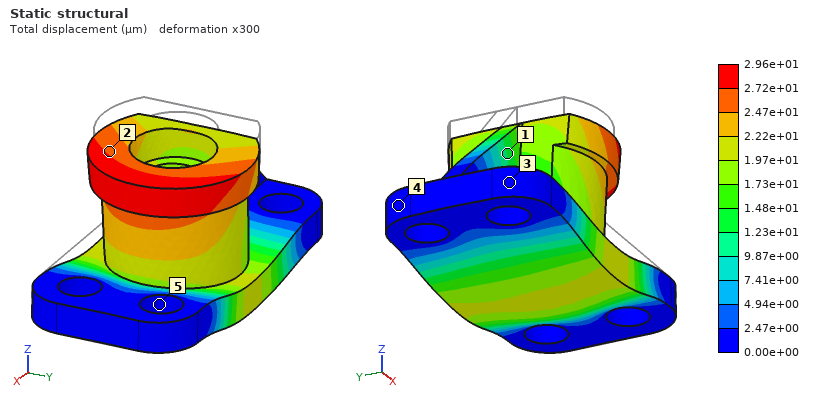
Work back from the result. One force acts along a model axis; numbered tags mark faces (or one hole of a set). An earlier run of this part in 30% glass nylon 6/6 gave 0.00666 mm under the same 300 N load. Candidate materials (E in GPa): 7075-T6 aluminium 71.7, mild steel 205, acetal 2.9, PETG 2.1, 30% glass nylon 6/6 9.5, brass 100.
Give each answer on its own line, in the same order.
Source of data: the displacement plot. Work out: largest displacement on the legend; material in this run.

2.96e+01 µm
PETG
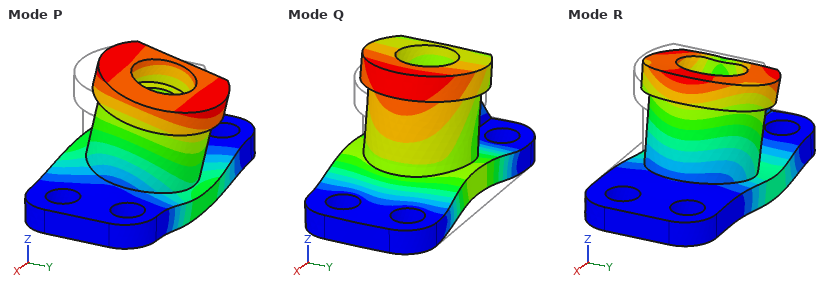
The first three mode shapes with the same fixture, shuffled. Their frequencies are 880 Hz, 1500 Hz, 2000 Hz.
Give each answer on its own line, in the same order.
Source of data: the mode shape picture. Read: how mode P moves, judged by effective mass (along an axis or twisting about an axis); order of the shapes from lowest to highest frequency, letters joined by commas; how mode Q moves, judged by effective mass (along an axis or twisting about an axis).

along Y
P, Q, R
along Z
